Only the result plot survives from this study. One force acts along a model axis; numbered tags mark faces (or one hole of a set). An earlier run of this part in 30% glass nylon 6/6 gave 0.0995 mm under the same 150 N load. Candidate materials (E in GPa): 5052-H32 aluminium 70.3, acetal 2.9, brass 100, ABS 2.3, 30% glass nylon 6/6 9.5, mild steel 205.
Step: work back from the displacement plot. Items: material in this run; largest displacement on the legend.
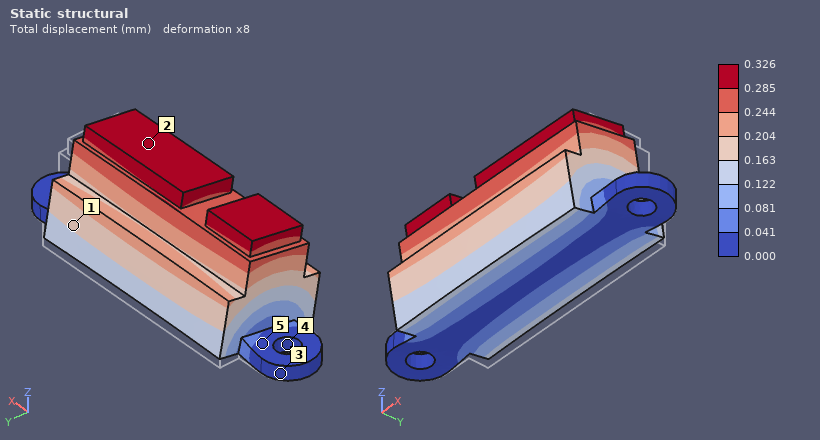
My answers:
acetal
0.326 mm
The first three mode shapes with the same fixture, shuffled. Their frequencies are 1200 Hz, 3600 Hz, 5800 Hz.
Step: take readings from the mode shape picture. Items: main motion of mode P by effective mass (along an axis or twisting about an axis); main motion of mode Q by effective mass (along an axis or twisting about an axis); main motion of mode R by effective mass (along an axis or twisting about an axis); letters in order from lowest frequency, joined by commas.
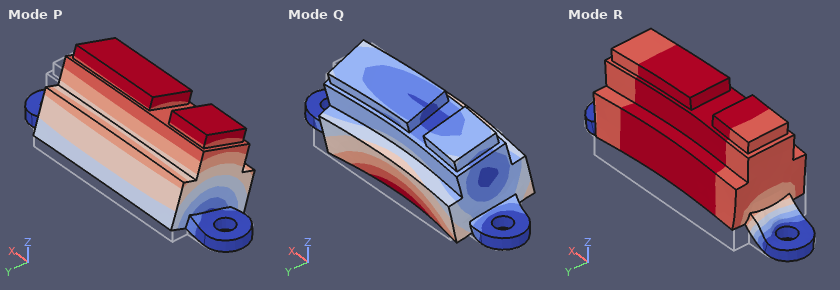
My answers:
along Y
along Y
along Z
P, R, Q
